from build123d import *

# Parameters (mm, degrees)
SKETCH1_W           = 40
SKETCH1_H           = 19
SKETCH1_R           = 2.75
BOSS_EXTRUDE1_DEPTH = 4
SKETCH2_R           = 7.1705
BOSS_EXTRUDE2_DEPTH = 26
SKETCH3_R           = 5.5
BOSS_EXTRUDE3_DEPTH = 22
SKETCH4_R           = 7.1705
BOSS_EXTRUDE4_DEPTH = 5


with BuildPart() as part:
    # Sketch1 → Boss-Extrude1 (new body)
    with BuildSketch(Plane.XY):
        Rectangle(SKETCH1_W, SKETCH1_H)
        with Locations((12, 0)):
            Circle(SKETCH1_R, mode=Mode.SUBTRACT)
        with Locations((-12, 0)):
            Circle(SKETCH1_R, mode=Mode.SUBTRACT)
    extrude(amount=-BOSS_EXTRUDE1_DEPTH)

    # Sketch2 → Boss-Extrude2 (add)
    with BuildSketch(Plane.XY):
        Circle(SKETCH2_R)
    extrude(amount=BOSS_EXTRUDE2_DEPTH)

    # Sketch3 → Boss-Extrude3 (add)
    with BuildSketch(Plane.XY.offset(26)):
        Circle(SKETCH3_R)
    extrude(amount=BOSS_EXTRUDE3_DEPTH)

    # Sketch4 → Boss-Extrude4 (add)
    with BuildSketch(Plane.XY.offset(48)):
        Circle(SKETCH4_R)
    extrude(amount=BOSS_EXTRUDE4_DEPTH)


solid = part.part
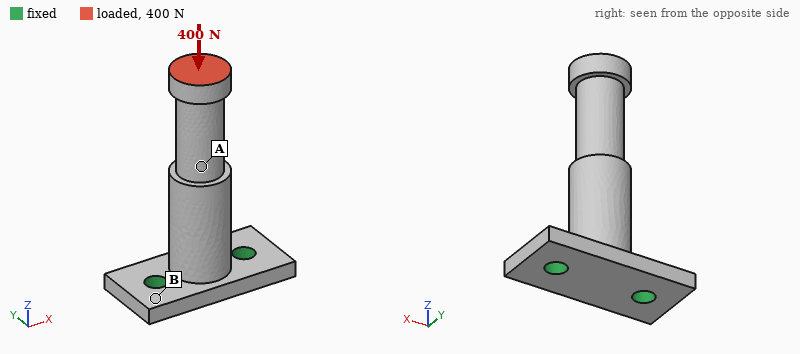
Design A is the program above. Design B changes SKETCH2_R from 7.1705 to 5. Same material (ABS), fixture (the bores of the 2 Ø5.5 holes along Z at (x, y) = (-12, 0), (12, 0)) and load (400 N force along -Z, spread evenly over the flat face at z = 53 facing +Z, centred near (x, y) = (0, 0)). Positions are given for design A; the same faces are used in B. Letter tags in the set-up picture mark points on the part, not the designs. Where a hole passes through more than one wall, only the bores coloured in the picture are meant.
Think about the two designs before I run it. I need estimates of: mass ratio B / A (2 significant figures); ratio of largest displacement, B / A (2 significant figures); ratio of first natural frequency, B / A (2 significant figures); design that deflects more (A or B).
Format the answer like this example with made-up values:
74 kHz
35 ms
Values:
0.78
1.5
0.73
B
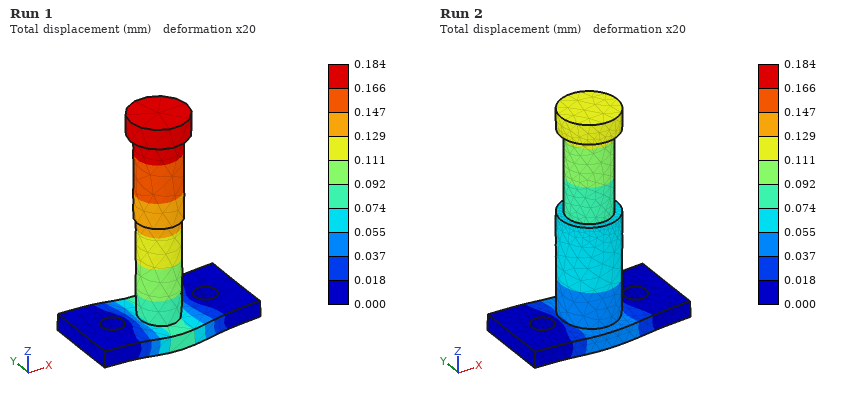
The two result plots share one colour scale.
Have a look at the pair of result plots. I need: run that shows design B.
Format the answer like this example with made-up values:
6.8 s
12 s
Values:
Run 1
